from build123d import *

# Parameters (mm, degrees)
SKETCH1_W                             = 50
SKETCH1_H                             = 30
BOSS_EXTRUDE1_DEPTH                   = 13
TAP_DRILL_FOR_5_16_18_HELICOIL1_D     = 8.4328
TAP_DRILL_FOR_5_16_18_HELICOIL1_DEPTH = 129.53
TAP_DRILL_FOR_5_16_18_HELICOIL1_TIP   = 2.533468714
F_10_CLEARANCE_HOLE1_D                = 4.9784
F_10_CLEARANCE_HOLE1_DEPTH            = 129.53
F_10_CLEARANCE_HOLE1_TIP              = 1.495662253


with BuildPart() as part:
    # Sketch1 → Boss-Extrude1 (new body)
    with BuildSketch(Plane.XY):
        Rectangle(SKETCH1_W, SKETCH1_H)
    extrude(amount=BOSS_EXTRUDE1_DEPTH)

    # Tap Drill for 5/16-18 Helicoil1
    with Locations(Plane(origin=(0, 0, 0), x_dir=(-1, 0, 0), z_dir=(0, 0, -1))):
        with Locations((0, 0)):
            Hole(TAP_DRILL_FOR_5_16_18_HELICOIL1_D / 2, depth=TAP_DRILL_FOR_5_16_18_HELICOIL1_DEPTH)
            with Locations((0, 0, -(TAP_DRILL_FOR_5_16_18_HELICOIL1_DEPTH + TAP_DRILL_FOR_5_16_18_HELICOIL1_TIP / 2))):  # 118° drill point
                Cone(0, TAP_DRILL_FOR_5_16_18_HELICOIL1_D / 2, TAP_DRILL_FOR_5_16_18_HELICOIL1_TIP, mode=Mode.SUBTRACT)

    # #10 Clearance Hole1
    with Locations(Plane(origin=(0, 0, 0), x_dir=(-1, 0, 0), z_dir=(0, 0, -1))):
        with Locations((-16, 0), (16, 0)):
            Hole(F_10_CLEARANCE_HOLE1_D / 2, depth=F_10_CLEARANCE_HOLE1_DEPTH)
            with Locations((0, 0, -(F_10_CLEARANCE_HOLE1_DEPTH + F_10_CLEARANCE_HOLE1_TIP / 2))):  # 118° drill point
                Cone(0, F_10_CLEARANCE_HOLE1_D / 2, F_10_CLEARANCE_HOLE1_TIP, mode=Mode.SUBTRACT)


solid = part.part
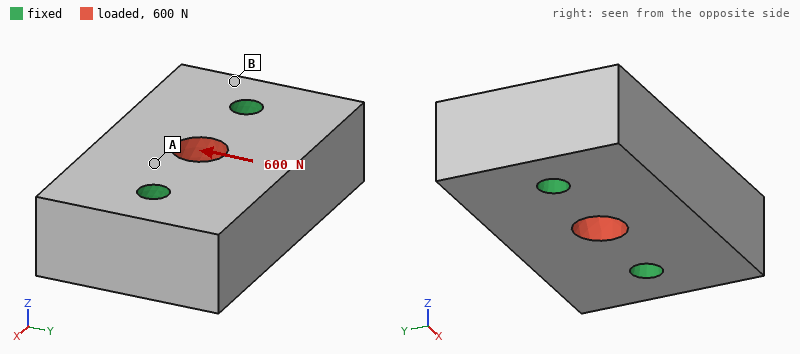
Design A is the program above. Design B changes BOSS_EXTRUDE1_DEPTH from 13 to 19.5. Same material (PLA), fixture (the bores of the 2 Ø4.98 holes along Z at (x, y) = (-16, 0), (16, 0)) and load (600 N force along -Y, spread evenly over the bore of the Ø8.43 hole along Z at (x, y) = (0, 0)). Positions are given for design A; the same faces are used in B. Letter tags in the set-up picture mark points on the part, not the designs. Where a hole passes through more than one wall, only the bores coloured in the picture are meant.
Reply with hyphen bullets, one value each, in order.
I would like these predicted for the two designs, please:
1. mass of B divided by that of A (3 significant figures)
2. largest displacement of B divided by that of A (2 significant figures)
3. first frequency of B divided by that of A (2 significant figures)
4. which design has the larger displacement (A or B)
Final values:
- 1.50
- 0.68
- 1.2
- A
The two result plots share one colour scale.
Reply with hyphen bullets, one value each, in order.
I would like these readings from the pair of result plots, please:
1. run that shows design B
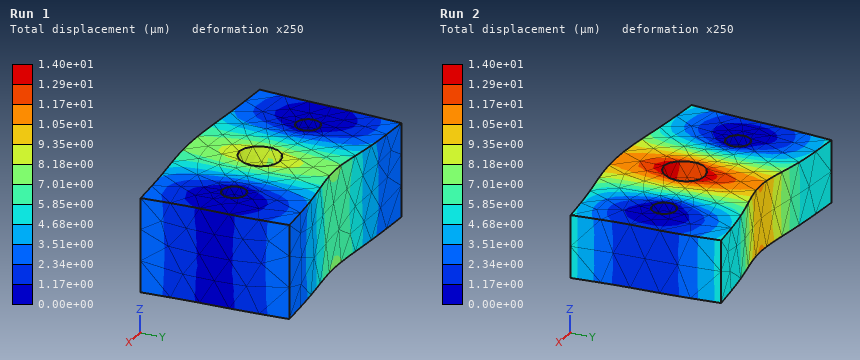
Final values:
- Run 1
